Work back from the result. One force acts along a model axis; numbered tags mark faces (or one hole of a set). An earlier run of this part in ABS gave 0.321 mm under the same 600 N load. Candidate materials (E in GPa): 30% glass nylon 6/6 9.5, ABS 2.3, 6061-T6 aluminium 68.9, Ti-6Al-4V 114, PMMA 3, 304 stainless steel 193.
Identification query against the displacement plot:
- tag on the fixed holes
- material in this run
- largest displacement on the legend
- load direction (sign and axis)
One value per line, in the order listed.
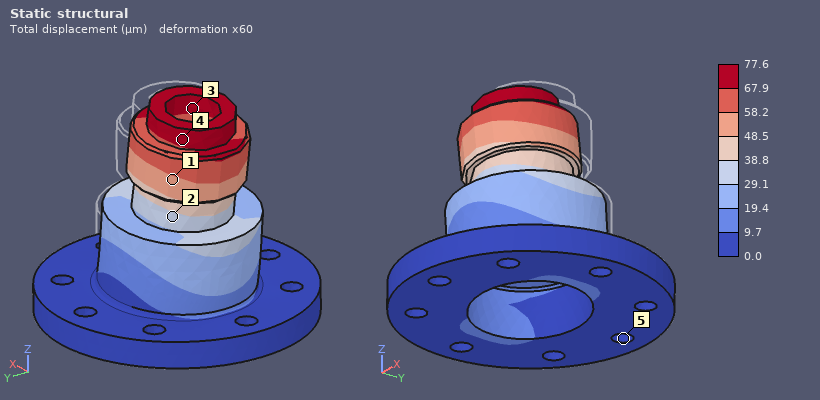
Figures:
5
30% glass nylon 6/6
77.6 µm
-X
